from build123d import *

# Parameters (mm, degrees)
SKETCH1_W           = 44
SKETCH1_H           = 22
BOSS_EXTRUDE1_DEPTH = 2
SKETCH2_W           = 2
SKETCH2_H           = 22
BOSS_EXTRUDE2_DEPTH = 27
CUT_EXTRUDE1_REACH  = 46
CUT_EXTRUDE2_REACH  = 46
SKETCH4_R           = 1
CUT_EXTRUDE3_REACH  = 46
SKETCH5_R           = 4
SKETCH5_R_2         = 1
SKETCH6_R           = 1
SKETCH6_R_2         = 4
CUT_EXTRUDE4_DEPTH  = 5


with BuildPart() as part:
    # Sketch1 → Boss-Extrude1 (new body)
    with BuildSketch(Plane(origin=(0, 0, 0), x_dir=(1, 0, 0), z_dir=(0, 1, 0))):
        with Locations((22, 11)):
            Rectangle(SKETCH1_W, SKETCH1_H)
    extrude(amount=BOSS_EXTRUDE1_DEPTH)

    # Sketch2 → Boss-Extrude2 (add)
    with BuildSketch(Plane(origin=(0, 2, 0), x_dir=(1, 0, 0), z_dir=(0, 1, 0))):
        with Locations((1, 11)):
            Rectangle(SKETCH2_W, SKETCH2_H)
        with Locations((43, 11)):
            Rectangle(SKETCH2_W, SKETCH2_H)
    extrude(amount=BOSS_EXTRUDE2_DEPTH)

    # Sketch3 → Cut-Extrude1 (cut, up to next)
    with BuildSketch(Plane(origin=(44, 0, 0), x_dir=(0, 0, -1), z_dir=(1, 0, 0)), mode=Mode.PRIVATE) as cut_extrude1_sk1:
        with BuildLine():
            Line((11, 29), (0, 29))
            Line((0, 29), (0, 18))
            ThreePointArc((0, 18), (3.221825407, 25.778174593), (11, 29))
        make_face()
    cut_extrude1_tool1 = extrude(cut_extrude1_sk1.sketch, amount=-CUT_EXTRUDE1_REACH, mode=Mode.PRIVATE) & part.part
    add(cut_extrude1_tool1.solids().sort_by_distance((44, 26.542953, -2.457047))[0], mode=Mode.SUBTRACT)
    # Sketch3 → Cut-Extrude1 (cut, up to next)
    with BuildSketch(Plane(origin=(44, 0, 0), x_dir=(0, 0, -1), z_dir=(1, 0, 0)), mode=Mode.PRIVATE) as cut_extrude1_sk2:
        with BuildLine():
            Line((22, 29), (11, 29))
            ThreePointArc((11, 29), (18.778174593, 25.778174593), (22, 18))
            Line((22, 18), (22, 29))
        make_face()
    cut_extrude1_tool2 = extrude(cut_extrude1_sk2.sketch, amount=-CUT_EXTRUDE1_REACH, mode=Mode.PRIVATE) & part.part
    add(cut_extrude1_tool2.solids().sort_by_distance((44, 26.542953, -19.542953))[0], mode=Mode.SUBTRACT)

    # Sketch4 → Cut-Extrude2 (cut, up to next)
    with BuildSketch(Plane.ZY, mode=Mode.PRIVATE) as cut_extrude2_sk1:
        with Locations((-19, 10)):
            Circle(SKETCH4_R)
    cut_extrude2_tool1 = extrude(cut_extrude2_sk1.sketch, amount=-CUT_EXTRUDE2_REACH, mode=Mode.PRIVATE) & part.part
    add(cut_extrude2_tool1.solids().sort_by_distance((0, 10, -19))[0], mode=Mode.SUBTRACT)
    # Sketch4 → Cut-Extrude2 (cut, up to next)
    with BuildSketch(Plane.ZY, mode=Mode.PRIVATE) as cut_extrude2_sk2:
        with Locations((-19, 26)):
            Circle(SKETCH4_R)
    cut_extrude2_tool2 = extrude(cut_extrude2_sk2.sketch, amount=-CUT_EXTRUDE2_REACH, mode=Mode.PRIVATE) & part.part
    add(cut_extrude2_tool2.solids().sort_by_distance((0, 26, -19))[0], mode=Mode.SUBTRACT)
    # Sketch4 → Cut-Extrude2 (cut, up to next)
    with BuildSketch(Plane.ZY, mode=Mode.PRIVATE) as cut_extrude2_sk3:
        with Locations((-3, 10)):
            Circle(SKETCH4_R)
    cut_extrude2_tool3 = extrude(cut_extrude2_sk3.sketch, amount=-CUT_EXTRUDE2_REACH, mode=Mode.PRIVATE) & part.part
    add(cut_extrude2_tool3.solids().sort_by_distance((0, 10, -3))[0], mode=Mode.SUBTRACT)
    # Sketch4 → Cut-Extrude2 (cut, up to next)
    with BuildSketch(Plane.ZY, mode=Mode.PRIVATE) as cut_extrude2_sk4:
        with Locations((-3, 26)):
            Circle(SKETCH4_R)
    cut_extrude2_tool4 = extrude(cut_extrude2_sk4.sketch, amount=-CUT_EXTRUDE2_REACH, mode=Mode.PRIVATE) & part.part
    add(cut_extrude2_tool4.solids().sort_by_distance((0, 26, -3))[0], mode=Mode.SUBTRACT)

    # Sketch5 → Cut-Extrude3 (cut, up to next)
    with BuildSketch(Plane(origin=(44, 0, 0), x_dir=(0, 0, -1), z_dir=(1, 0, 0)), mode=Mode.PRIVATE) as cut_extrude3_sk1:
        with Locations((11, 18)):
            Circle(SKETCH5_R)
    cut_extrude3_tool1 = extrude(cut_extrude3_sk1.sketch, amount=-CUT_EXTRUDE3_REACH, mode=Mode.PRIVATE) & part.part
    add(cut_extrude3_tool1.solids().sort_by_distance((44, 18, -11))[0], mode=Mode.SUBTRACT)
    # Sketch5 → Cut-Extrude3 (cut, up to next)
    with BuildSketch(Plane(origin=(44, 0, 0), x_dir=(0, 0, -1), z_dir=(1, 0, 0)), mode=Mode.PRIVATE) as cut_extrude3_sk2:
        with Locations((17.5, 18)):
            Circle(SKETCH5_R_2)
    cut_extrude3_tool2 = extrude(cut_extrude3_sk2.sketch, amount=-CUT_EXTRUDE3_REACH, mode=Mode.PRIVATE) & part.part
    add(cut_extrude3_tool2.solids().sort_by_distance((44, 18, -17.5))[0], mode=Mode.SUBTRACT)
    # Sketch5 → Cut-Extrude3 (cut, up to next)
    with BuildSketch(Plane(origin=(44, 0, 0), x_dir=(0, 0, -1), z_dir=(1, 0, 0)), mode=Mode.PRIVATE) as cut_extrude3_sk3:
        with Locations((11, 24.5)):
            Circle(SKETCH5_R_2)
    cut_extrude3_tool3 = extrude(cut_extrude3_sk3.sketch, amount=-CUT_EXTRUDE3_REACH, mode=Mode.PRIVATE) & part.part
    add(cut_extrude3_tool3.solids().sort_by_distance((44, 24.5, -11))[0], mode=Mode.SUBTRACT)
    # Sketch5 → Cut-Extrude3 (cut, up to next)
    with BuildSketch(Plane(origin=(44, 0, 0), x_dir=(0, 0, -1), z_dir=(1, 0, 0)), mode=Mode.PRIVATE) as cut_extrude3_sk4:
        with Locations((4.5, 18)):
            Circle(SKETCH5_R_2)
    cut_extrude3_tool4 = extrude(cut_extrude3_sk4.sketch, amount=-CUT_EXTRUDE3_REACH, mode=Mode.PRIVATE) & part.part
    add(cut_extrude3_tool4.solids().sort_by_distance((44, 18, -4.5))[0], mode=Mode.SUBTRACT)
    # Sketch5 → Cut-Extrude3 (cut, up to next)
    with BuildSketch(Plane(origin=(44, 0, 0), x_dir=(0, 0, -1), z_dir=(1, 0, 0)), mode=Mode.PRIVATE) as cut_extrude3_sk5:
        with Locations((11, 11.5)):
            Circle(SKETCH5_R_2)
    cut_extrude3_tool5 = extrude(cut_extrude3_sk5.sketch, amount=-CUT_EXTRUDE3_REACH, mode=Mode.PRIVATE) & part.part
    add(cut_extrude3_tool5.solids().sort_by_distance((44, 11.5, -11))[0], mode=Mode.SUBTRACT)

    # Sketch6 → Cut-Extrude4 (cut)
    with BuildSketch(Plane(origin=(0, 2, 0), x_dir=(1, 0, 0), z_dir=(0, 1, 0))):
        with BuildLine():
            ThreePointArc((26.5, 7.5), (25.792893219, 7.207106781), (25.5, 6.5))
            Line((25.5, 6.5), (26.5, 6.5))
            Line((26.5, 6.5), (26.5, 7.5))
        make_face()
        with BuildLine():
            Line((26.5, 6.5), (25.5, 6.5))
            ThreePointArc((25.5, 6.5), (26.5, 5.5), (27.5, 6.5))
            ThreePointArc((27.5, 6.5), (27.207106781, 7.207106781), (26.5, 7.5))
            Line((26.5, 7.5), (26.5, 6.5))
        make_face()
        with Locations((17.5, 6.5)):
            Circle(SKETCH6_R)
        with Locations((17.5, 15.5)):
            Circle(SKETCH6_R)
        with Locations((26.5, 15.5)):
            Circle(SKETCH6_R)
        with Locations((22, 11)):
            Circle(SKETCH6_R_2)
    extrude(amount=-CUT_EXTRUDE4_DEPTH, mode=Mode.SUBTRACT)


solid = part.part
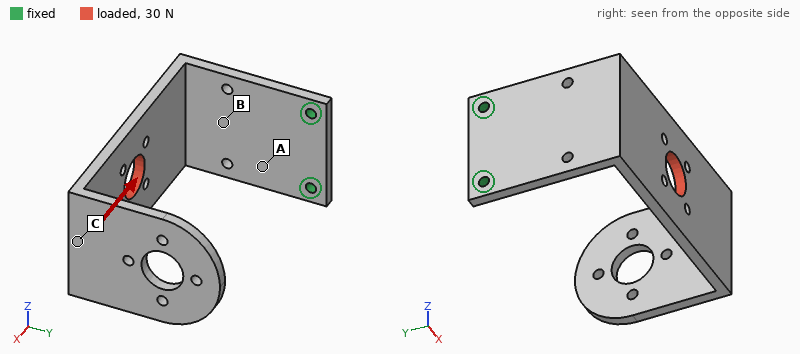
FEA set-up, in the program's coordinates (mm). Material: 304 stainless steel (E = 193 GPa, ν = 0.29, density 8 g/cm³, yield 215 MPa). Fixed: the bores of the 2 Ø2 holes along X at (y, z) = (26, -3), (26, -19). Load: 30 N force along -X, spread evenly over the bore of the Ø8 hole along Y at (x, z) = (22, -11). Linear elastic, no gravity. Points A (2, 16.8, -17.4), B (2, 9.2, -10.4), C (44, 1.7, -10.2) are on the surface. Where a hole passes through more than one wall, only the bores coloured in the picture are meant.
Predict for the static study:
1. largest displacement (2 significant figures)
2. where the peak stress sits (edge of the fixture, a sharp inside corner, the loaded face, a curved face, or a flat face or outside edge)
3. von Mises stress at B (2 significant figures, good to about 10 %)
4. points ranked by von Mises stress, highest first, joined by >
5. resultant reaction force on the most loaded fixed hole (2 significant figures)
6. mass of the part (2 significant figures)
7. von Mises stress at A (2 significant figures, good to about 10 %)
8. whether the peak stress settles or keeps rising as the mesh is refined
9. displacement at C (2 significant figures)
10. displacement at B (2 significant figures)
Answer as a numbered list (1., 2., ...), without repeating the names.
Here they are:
1. 0.16 mm
2. edge of the fixture
3. 18 MPa
4. A > B > C
5. 15 N
6. 31 g
7. 31 MPa
8. keeps rising
9. 0.16 mm
10. 0.032 mm
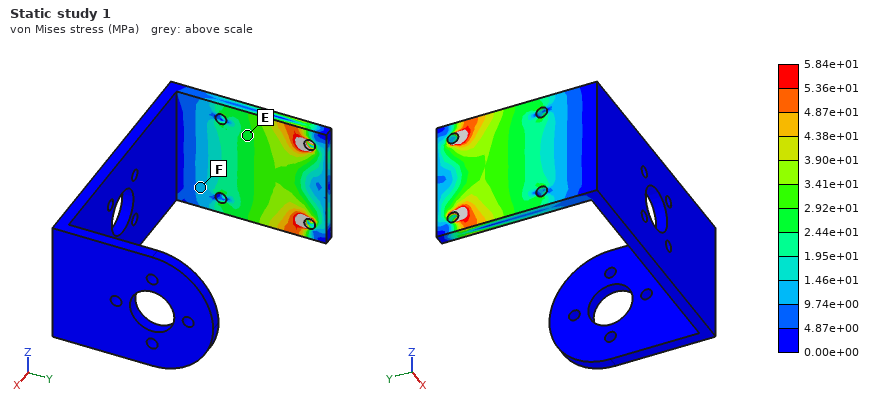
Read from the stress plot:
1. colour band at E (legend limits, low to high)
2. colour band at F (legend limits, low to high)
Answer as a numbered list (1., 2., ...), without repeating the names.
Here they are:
1. 2.44e+01 to 2.92e+01 MPa
2. 9.74e+00 to 1.46e+01 MPa
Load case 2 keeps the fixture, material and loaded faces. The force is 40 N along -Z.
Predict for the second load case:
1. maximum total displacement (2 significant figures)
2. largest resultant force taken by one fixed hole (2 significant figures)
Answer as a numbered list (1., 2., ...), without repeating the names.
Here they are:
1. 0.17 mm
2. 80 N
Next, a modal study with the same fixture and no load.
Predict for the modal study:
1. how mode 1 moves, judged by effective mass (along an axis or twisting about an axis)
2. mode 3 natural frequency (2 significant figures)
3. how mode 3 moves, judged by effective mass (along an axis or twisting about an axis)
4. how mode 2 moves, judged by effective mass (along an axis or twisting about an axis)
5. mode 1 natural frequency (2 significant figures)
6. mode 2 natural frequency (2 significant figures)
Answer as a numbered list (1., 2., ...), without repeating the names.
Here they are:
1. along Y
2. 830 Hz
3. along X
4. along Z
5. 280 Hz
6. 470 Hz
